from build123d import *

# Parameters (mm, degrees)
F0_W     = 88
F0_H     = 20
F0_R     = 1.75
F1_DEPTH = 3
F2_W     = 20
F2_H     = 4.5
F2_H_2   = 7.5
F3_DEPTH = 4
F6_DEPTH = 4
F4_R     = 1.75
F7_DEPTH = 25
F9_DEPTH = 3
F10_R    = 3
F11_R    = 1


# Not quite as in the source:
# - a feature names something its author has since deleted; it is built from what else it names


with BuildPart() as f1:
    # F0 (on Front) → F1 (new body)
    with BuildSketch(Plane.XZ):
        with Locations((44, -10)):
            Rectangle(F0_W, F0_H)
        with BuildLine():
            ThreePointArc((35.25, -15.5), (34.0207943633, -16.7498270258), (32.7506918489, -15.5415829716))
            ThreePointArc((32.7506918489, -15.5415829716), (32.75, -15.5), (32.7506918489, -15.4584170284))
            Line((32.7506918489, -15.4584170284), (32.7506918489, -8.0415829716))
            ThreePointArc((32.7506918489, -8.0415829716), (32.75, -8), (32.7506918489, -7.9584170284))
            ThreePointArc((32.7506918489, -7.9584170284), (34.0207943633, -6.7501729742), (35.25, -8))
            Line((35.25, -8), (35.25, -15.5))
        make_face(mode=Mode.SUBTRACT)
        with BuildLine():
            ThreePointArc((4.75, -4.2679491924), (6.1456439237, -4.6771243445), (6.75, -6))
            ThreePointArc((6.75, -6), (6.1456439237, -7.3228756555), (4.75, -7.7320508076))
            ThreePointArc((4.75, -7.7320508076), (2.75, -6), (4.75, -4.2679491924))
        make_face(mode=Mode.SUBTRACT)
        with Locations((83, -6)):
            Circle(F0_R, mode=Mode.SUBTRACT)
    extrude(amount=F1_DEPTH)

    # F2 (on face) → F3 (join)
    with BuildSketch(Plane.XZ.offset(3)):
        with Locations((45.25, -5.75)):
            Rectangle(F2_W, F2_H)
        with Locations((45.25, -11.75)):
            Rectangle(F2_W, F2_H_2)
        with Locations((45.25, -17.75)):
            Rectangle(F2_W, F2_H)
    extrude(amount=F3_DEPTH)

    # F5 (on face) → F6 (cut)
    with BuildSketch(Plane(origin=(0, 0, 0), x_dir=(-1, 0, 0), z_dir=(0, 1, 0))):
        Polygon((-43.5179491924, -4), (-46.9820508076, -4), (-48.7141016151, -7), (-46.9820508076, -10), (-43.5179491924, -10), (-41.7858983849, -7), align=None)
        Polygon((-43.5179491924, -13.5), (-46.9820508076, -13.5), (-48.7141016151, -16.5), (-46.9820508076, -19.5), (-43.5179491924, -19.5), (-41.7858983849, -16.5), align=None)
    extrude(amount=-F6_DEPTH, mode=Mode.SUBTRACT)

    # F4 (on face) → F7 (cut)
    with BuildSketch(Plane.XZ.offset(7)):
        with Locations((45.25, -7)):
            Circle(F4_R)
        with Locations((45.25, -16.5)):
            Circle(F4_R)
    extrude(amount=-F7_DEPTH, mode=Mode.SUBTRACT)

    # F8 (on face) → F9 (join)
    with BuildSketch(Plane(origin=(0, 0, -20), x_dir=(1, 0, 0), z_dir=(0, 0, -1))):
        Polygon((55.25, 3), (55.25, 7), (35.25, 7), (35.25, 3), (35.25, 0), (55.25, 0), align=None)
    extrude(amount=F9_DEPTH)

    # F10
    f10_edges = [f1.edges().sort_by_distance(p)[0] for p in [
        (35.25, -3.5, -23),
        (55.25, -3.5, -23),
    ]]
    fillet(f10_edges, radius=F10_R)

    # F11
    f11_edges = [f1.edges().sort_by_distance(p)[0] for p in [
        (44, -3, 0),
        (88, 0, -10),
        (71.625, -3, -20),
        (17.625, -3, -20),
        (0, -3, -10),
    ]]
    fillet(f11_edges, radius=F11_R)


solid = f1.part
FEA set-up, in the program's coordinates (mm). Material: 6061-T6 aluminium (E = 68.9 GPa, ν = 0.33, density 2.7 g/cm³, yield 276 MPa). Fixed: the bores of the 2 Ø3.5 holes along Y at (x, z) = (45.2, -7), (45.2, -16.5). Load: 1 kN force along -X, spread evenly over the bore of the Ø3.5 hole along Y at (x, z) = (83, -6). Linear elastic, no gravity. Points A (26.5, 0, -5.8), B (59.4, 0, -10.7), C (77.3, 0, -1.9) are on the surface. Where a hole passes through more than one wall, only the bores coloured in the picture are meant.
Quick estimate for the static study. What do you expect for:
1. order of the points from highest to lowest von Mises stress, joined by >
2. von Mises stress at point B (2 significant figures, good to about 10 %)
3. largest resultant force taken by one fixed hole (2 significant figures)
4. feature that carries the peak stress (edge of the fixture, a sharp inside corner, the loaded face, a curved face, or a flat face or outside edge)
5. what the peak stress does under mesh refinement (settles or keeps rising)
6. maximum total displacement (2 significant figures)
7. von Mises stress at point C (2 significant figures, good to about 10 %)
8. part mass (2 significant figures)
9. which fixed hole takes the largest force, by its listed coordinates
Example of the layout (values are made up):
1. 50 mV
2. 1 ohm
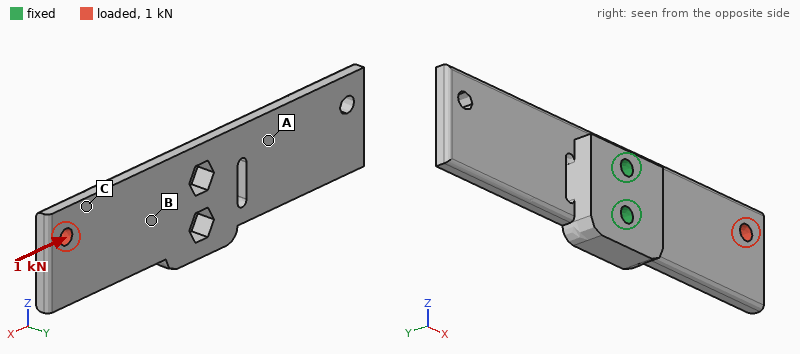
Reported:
1. C > B > A
2. 17 MPa
3. 990 N
4. edge of the fixture
5. keeps rising
6. 85 µm
7. 30 MPa
8. 18 g
9. (45.2, -7)
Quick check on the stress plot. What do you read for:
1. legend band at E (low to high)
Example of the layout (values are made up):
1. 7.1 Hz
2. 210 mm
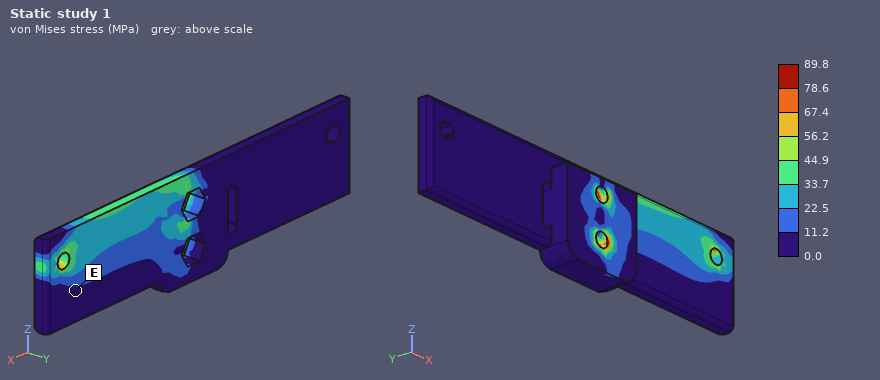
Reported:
1. 0.0 to 11.2 MPa
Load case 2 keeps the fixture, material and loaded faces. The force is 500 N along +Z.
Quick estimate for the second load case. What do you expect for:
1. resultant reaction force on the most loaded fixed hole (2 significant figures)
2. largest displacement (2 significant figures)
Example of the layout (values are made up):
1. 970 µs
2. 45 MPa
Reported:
1. 1.6 kN
2. 0.11 mm
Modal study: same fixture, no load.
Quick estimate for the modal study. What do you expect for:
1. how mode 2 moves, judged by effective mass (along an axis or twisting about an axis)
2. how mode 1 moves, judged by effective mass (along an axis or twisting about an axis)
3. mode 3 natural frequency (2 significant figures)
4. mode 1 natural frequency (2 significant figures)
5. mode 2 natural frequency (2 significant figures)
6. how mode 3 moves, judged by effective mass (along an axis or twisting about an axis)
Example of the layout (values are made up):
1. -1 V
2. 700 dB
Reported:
1. along Y
2. along Y
3. 5900 Hz
4. 1400 Hz
5. 1900 Hz
6. twisting about Y
